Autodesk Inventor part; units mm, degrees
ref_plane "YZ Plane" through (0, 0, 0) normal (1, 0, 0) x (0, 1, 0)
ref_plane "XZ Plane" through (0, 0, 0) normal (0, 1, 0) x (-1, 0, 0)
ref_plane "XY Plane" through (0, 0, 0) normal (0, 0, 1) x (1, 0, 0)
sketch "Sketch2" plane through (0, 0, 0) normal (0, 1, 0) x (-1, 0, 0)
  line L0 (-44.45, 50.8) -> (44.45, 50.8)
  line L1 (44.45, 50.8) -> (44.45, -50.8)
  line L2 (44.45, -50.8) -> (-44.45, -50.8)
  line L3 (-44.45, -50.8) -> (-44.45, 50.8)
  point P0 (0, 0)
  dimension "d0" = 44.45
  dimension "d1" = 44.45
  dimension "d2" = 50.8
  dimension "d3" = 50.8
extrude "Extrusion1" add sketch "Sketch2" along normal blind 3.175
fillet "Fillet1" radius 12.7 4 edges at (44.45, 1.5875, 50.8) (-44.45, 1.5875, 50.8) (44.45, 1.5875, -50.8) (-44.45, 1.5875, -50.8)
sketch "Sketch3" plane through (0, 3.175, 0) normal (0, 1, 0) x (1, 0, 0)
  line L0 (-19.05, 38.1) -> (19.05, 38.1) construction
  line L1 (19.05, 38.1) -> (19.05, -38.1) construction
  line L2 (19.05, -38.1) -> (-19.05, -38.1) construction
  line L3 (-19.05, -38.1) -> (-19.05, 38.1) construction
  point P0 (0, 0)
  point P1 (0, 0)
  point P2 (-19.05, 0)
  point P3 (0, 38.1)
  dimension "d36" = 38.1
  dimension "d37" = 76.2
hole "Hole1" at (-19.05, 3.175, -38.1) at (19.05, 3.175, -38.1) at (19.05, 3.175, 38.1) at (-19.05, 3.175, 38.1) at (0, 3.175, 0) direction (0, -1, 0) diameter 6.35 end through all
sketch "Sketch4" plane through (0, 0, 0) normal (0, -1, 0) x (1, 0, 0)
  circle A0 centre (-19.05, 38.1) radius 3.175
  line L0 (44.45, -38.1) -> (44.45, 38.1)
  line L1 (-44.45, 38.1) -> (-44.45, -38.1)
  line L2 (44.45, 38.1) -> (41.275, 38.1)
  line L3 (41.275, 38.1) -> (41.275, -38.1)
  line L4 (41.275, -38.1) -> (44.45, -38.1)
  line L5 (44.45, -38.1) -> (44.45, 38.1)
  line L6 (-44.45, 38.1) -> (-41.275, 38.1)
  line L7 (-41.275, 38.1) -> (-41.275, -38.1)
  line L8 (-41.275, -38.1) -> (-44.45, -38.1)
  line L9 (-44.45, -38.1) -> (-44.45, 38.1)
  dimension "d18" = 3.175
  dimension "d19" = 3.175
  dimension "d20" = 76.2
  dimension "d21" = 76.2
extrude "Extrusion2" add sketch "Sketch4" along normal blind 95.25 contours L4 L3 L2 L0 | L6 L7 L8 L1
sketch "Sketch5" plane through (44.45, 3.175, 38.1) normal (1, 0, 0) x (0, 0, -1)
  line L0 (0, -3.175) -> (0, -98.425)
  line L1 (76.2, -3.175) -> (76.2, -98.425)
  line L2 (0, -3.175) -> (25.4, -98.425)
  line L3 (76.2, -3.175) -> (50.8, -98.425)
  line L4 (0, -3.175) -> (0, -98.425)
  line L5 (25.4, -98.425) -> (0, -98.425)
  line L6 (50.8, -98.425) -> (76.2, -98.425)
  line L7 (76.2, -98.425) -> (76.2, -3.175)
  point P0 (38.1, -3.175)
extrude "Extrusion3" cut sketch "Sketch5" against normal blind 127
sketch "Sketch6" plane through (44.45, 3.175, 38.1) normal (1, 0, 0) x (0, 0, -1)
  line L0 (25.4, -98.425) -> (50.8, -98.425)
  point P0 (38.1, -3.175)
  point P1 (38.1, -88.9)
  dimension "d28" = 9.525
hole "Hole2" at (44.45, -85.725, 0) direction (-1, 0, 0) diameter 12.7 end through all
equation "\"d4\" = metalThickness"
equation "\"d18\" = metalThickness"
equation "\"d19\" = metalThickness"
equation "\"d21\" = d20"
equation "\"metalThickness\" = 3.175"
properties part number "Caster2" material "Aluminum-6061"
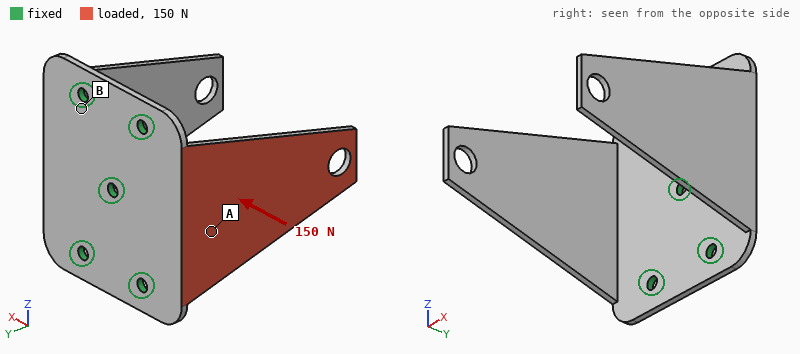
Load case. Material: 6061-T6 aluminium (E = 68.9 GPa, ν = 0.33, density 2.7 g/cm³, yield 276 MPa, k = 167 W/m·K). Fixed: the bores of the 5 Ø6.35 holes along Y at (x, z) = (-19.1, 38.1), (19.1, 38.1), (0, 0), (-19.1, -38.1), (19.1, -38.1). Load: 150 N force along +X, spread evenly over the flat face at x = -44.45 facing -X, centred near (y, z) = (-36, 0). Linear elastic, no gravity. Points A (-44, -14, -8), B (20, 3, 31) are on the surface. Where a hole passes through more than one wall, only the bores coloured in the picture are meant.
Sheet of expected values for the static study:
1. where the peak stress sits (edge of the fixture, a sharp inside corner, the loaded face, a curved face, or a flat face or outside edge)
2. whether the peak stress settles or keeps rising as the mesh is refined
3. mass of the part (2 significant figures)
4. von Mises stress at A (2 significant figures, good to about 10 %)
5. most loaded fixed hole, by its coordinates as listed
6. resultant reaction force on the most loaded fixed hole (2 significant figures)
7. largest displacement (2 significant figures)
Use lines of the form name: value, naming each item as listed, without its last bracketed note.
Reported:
where the peak stress sits: edge of the fixture
whether the peak stress settles or keeps rising as the mesh is refined: keeps rising
mass of the part: 160 g
von Mises stress at A: 28 MPa
most loaded fixed hole, by its coordinates as listed: (0, 0)
resultant reaction force on the most loaded fixed hole: 130 N
largest displacement: 1.6 mm
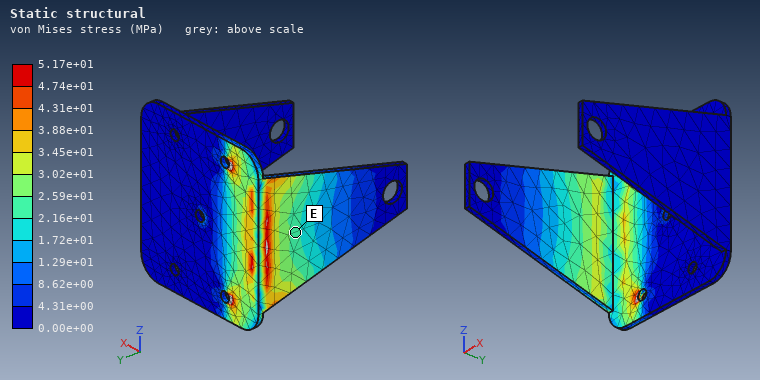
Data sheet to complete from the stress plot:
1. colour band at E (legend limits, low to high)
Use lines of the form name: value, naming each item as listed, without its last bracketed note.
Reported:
colour band at E: 2.16e+01 to 2.59e+01 MPa
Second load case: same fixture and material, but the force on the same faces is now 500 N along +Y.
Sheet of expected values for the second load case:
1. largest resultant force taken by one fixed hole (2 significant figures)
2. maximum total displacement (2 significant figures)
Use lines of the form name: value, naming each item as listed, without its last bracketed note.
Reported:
largest resultant force taken by one fixed hole: 300 N
maximum total displacement: 1.0 mm
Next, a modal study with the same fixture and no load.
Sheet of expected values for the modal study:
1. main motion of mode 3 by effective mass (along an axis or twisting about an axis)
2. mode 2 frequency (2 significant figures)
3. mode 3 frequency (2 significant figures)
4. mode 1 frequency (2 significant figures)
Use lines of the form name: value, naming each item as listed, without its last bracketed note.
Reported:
main motion of mode 3 by effective mass: along Z
mode 2 frequency: 310 Hz
mode 3 frequency: 1100 Hz
mode 1 frequency: 310 Hz
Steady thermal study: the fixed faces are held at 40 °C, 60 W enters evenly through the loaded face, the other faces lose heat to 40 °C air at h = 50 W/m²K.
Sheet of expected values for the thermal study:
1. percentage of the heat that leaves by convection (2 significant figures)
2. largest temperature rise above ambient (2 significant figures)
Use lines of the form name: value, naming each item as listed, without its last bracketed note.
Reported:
percentage of the heat that leaves by convection: 34 %
largest temperature rise above ambient: 75 K
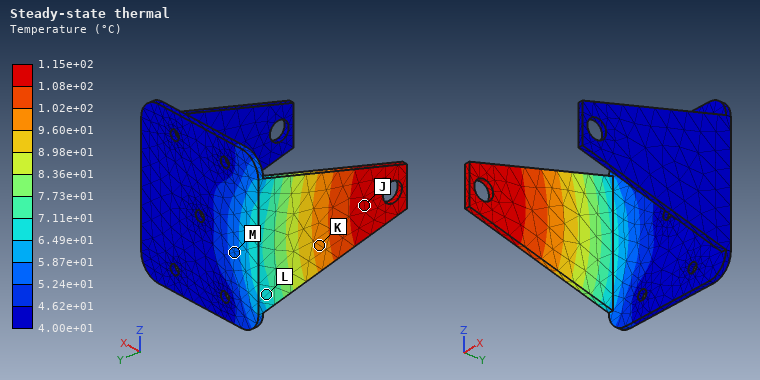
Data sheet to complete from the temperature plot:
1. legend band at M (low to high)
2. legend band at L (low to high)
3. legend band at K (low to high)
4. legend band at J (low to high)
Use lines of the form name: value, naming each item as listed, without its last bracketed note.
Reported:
legend band at M: 5.24e+01 to 5.87e+01 °C
legend band at L: 6.49e+01 to 7.11e+01 °C
legend band at K: 9.60e+01 to 1.02e+02 °C
legend band at J: 1.08e+02 to 1.15e+02 °C
